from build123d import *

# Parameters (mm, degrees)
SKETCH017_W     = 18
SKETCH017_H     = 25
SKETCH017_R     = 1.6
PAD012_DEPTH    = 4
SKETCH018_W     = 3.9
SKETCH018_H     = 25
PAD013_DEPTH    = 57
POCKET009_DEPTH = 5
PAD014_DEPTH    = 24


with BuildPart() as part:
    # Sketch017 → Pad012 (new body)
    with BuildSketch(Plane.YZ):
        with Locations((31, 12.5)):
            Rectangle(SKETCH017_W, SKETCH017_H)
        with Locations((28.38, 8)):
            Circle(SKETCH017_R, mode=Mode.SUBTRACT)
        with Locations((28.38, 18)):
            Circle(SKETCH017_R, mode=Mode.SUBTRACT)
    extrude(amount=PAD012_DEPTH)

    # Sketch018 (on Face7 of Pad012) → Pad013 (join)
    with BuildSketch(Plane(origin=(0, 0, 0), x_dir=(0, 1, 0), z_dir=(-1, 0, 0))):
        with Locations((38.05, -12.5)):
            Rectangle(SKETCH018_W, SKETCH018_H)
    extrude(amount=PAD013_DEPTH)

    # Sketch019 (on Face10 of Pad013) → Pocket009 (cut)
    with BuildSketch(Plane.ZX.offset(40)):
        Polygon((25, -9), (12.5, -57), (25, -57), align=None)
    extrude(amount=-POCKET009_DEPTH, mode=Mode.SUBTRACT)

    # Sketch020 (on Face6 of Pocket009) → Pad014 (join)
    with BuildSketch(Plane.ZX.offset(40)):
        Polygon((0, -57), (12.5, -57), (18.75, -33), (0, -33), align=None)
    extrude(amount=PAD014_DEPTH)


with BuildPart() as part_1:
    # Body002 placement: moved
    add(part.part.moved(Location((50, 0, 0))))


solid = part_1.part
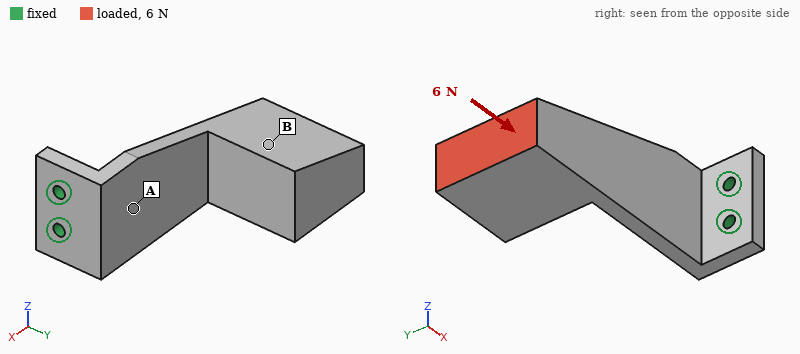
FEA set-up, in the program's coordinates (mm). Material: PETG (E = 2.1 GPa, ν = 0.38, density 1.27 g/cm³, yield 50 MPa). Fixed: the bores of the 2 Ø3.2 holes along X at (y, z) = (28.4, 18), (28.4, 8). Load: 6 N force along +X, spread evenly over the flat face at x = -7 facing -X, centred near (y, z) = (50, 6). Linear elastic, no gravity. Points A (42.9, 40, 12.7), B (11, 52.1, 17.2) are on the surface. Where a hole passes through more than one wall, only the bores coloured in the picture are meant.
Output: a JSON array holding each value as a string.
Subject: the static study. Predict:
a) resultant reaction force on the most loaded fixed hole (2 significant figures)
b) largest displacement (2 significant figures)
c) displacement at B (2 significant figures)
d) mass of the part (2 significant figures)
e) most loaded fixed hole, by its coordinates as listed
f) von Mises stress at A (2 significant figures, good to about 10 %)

["5.7 N", "0.73 mm", "0.41 mm", "19 g", "(28.4, 8)", "1.1 MPa"]
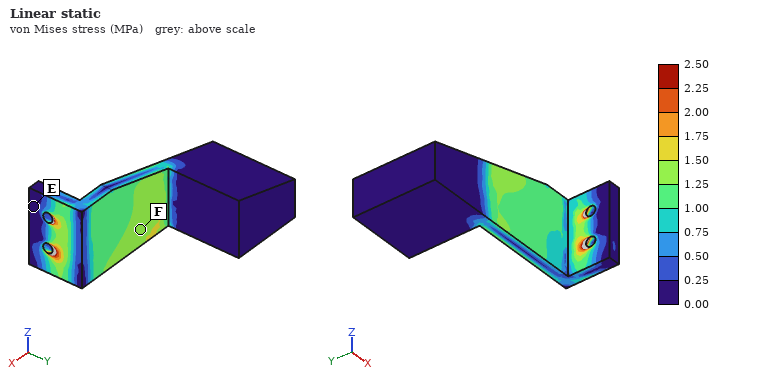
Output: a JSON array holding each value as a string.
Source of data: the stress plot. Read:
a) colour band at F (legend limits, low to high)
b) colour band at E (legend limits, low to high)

["1.25 to 1.50 MPa", "0.00 to 0.25 MPa"]
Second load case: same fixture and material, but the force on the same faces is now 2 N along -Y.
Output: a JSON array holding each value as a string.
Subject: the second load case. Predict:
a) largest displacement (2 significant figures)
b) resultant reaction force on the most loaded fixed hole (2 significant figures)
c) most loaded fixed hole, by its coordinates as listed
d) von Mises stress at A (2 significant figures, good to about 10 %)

["0.83 mm", "2.6 N", "(28.4, 8)", "1.4 MPa"]
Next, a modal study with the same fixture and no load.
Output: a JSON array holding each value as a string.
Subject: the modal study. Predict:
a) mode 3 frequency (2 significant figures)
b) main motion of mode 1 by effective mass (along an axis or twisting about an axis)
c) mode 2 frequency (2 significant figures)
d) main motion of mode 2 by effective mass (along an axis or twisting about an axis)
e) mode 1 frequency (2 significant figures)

["510 Hz", "along Y", "230 Hz", "along Z", "90 Hz"]
